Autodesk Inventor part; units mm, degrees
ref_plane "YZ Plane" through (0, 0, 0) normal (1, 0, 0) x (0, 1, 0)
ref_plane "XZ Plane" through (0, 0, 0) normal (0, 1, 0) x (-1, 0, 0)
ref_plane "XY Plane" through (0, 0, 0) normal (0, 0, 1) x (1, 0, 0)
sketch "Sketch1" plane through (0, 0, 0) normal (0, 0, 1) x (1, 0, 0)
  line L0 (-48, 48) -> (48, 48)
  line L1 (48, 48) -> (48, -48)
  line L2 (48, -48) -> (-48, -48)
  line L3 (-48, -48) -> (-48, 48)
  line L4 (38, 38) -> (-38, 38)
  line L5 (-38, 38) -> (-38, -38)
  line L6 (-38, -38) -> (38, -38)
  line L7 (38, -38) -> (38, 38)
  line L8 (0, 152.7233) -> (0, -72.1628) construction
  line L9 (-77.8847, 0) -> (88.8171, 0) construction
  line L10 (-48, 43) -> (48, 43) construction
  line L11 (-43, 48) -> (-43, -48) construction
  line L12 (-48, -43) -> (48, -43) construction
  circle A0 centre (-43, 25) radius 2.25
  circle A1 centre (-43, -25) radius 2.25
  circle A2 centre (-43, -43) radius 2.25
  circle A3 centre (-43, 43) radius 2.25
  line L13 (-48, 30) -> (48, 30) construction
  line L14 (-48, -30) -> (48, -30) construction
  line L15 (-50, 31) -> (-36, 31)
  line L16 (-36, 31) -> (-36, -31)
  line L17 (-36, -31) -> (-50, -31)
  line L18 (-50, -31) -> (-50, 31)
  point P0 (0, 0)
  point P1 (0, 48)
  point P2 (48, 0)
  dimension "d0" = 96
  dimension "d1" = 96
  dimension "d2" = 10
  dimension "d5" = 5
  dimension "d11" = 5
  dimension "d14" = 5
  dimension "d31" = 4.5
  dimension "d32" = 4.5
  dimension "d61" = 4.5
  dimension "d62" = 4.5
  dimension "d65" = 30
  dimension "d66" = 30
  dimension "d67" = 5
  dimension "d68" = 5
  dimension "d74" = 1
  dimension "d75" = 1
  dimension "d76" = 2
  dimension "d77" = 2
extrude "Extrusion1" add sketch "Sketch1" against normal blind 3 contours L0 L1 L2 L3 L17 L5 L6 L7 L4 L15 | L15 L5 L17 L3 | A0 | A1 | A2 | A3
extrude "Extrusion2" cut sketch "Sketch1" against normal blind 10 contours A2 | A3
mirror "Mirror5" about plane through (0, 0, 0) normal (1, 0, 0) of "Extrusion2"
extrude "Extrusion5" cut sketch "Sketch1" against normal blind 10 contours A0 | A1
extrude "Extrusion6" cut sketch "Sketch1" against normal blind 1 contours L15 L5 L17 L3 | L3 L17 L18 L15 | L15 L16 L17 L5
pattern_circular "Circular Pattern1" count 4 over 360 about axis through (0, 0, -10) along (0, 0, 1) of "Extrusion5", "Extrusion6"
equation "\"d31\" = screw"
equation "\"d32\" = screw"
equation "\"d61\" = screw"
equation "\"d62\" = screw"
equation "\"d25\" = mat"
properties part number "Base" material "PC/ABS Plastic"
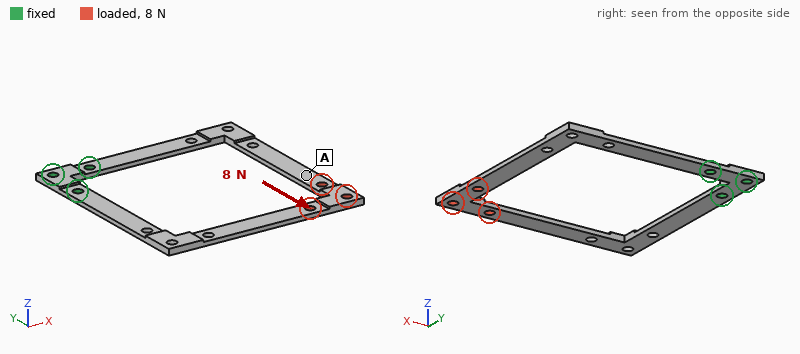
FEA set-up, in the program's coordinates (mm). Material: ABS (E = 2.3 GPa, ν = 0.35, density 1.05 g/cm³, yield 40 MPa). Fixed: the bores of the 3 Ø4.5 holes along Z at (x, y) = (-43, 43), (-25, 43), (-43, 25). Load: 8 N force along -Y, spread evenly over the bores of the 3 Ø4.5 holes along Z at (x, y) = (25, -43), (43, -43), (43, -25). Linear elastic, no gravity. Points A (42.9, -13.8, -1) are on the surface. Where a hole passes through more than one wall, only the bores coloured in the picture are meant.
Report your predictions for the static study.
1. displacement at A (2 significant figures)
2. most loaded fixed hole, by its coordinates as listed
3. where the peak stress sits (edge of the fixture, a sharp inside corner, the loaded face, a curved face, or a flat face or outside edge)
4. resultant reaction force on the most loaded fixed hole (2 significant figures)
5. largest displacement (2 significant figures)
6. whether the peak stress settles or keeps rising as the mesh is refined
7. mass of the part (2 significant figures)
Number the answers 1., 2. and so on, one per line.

1. 1.2 mm
2. (-25, 43)
3. edge of the fixture
4. 12 N
5. 1.4 mm
6. keeps rising
7. 7.8 g
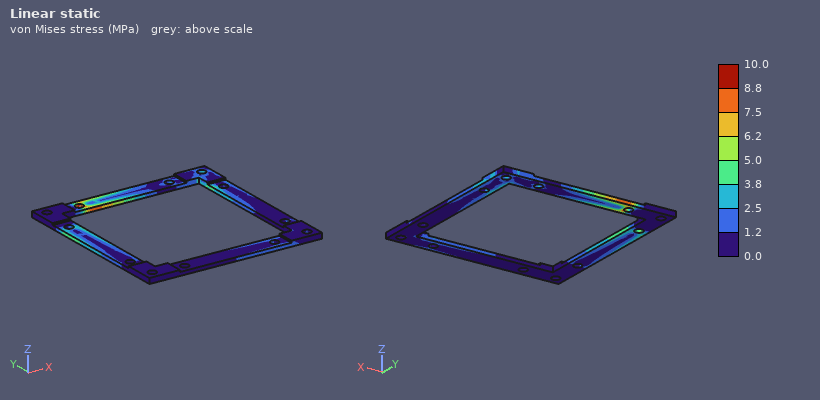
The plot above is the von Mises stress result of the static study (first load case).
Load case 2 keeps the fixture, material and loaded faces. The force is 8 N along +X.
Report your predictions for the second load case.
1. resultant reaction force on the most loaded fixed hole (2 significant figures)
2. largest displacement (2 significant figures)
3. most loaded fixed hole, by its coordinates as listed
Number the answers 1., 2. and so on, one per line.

1. 12 N
2. 1.4 mm
3. (-43, 25)
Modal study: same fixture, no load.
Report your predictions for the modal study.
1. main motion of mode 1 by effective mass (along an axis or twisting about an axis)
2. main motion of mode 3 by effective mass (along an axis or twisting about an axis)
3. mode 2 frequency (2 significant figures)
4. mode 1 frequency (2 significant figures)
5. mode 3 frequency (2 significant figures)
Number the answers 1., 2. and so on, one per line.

1. along Z
2. along Z
3. 63 Hz
4. 29 Hz
5. 120 Hz
